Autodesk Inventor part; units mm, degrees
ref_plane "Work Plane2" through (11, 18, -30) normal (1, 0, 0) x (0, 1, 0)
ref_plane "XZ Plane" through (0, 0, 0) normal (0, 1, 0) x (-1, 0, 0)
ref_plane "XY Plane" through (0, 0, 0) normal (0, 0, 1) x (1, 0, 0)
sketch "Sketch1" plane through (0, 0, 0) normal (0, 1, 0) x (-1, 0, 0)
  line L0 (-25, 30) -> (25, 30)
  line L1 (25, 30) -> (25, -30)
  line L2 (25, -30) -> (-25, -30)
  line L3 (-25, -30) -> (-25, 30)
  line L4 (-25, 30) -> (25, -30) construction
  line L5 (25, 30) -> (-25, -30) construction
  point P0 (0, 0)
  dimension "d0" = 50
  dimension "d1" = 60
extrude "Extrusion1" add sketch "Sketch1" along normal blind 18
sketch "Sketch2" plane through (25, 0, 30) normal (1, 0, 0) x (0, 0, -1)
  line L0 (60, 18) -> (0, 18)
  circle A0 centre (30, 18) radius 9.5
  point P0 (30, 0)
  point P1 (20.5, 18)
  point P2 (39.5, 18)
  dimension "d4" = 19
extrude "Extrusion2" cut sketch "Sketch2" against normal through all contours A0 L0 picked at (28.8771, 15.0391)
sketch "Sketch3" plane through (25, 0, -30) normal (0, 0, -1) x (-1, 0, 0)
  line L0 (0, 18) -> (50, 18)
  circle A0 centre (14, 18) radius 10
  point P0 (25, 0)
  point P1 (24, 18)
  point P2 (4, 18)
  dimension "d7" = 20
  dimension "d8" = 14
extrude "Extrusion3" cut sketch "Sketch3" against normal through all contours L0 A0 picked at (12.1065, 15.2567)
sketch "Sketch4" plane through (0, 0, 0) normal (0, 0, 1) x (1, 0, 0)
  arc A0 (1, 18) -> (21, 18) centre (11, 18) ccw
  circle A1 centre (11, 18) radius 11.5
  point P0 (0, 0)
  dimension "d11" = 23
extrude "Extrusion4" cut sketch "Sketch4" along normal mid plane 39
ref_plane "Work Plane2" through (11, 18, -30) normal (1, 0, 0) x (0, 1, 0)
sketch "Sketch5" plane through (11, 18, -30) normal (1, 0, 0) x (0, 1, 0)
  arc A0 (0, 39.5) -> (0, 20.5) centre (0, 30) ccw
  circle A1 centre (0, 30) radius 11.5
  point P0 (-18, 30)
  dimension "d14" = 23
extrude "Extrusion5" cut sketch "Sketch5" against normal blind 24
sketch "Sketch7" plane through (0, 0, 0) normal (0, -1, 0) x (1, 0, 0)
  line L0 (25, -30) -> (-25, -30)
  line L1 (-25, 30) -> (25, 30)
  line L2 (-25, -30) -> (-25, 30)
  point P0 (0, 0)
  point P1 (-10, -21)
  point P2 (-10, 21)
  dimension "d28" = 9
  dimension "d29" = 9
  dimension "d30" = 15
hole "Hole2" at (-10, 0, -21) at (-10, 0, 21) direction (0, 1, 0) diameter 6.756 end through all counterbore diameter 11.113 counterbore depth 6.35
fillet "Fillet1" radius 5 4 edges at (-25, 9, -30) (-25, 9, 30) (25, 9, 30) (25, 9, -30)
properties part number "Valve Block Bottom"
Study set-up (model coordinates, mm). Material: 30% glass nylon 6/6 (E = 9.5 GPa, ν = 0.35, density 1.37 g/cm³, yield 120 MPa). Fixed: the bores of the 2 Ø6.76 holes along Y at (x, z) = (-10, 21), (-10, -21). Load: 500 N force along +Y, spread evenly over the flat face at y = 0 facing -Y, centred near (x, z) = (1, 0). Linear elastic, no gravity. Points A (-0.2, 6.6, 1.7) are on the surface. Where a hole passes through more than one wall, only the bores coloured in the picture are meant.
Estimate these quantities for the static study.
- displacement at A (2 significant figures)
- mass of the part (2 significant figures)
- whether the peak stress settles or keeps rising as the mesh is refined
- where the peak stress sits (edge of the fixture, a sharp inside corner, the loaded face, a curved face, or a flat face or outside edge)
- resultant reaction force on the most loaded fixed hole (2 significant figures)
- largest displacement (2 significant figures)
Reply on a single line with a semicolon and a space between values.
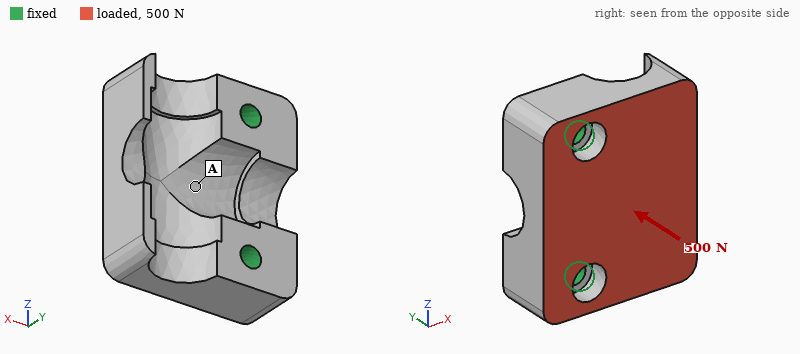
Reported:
8.7 µm; 48 g; keeps rising; edge of the fixture; 270 N; 49 µm
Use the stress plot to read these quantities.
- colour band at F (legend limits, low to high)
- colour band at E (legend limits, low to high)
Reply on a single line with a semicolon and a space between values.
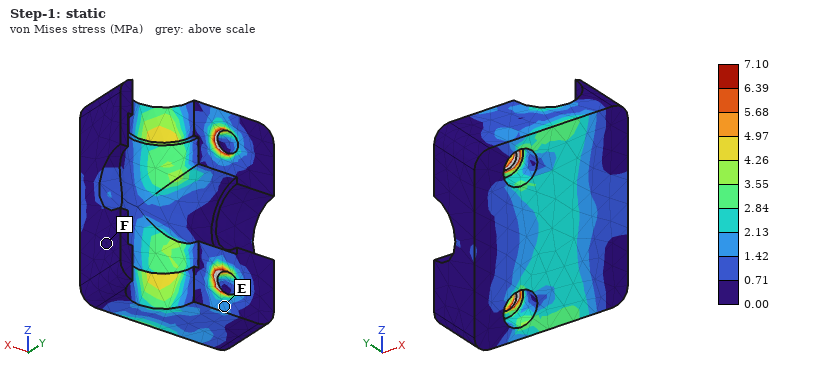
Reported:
0.00 to 0.71 MPa; 1.42 to 2.13 MPa
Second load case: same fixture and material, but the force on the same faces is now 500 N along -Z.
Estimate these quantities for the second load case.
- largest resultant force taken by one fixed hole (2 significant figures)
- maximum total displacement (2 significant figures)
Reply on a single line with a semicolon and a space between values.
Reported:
290 N; 8.3 µm
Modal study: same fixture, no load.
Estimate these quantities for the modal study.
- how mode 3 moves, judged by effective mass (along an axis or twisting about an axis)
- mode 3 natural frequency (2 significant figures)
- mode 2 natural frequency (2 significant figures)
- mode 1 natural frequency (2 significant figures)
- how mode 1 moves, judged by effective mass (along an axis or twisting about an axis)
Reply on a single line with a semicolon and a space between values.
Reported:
along Z; 7700 Hz; 4500 Hz; 3100 Hz; along Y
